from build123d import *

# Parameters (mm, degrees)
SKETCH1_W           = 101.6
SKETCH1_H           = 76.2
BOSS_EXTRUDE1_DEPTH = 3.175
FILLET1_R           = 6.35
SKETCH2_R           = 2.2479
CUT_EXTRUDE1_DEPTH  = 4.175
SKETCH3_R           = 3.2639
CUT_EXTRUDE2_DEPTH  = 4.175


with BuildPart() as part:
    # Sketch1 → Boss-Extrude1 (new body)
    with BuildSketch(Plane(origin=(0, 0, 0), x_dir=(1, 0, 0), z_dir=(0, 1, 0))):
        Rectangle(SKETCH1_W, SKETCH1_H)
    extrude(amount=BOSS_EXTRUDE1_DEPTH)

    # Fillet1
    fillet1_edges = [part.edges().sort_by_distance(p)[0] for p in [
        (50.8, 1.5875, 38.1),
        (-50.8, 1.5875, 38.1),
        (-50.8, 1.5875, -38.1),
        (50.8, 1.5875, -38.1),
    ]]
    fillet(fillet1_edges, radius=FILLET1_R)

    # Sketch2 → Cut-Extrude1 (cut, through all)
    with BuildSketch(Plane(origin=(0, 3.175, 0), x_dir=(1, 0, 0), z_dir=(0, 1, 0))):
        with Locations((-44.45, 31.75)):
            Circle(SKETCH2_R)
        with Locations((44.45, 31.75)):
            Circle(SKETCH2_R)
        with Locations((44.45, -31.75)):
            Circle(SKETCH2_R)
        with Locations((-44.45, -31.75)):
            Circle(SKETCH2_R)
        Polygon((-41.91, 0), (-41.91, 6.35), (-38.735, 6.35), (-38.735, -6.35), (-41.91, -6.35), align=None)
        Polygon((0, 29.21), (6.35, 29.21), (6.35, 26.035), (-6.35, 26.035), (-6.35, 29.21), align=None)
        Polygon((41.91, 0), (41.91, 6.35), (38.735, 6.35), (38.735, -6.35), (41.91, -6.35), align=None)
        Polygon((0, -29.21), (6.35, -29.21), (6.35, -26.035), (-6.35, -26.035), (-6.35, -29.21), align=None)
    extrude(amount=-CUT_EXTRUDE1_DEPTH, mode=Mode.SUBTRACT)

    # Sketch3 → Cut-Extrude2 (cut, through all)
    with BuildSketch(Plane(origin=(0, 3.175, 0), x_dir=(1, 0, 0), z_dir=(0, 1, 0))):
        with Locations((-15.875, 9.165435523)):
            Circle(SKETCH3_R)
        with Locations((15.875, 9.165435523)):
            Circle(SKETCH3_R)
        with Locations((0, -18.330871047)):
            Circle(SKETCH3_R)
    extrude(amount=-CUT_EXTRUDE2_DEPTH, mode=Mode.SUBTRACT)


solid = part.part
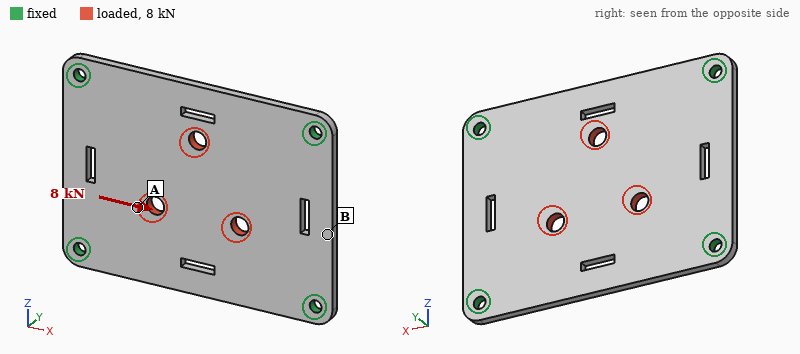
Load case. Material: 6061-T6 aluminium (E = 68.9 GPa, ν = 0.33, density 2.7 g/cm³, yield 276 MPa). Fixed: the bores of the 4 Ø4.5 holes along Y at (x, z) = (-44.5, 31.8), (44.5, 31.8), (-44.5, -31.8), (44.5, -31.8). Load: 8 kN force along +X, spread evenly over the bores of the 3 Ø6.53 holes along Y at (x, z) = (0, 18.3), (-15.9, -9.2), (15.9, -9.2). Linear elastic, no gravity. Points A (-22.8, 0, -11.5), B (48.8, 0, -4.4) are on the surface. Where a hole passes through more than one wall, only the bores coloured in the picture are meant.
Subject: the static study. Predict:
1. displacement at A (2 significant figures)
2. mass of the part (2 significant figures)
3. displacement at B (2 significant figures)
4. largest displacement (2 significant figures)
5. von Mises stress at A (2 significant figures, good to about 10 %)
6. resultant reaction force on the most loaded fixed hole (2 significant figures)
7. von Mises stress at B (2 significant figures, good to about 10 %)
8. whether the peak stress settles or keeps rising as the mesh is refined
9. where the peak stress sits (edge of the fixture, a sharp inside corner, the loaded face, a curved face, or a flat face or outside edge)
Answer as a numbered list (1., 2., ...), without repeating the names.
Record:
1. 20 µm
2. 63 g
3. 17 µm
4. 24 µm
5. 34 MPa
6. 2.2 kN
7. 15 MPa
8. keeps rising
9. edge of the fixture
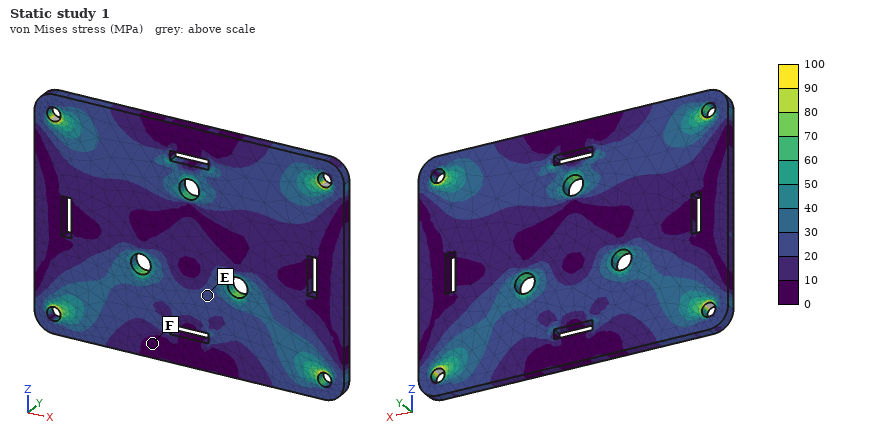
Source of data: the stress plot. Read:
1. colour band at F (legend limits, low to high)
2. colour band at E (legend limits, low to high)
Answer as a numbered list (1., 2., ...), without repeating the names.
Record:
1. 0 to 10 MPa
2. 20 to 30 MPa
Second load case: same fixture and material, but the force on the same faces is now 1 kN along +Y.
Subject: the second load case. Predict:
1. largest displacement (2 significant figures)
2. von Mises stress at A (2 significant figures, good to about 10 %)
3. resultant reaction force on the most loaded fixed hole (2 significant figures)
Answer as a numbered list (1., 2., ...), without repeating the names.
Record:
1. 0.38 mm
2. 50 MPa
3. 250 N
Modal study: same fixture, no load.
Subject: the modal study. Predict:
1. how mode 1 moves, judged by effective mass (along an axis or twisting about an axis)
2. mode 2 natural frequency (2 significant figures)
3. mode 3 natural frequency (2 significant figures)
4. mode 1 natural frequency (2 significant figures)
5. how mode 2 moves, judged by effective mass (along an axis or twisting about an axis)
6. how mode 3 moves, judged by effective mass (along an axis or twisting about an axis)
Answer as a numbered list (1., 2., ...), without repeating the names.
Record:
1. along Y
2. 2700 Hz
3. 3900 Hz
4. 1700 Hz
5. twisting about X
6. twisting about Z
